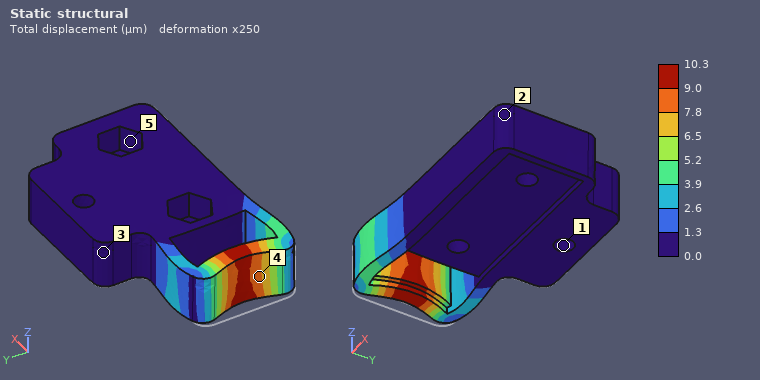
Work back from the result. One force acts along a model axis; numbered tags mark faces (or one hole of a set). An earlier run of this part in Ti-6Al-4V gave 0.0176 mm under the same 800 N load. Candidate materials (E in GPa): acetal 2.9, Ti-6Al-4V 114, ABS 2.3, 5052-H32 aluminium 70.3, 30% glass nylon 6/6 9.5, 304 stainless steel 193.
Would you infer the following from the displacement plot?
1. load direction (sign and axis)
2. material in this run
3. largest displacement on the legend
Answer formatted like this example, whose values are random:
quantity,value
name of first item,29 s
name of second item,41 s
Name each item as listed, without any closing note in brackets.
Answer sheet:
quantity,value
load direction,+X
material in this run,304 stainless steel
largest displacement on the legend,10.3 µm
